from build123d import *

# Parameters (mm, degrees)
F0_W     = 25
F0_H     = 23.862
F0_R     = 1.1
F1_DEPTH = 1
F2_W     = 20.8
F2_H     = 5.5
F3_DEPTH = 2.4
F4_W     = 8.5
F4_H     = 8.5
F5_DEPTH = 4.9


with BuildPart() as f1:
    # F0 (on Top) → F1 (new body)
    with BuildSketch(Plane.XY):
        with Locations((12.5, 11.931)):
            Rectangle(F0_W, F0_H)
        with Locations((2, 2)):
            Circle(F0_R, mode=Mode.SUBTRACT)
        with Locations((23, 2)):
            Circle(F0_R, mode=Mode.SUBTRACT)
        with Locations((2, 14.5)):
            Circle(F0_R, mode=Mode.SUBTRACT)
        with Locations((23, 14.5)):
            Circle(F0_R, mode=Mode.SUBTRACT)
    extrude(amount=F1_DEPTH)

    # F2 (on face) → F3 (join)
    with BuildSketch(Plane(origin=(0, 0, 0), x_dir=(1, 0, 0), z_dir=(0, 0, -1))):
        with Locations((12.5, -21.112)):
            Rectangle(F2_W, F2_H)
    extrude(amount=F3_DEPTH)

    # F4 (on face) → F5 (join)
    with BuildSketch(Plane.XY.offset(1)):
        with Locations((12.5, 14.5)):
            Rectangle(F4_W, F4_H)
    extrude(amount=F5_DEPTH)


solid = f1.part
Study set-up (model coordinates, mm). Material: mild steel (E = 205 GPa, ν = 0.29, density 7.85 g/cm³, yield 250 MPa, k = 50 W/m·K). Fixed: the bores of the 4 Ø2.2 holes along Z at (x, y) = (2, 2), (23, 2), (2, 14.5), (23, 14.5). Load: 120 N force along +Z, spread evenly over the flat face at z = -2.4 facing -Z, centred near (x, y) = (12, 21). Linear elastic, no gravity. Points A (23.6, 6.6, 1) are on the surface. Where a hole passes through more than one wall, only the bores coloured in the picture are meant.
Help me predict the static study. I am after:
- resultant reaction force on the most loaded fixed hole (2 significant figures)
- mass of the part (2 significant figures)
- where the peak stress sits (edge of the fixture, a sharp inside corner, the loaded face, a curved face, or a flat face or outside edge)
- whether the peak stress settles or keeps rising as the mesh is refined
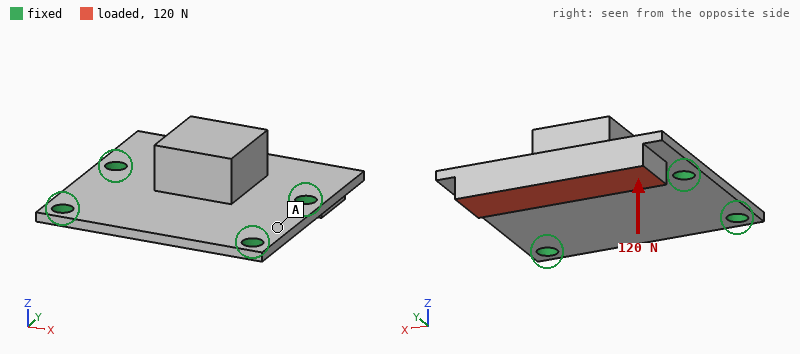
74 N
9.5 g
edge of the fixture
keeps rising
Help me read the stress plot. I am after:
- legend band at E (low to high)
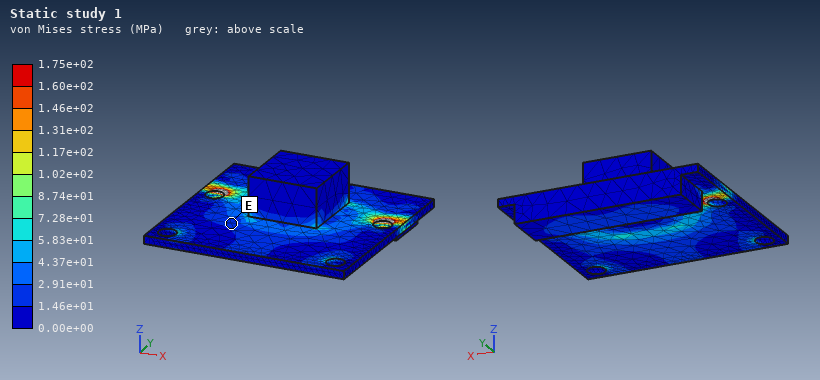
1.46e+01 to 2.91e+01 MPa
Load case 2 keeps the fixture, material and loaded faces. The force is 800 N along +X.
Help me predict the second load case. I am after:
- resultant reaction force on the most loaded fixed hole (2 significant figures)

450 N
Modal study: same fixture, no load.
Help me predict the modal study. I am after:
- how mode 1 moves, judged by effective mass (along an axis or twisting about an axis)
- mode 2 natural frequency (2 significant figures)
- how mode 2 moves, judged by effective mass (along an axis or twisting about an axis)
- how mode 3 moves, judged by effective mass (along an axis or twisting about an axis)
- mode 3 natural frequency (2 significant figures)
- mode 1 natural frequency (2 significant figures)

along Z
11 kHz
along Z
twisting about Y
18 kHz
6200 Hz
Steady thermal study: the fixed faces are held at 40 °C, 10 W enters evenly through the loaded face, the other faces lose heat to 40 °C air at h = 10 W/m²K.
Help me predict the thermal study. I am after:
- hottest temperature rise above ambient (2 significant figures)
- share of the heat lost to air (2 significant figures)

57 K
3.6 %
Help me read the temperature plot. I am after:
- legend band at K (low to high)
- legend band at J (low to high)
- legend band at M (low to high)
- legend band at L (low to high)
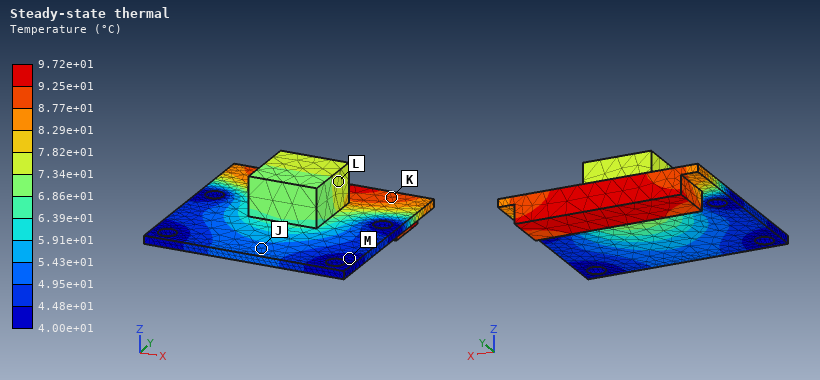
8.77e+01 to 9.25e+01 °C
4.95e+01 to 5.43e+01 °C
4.00e+01 to 4.48e+01 °C
7.34e+01 to 7.82e+01 °C
